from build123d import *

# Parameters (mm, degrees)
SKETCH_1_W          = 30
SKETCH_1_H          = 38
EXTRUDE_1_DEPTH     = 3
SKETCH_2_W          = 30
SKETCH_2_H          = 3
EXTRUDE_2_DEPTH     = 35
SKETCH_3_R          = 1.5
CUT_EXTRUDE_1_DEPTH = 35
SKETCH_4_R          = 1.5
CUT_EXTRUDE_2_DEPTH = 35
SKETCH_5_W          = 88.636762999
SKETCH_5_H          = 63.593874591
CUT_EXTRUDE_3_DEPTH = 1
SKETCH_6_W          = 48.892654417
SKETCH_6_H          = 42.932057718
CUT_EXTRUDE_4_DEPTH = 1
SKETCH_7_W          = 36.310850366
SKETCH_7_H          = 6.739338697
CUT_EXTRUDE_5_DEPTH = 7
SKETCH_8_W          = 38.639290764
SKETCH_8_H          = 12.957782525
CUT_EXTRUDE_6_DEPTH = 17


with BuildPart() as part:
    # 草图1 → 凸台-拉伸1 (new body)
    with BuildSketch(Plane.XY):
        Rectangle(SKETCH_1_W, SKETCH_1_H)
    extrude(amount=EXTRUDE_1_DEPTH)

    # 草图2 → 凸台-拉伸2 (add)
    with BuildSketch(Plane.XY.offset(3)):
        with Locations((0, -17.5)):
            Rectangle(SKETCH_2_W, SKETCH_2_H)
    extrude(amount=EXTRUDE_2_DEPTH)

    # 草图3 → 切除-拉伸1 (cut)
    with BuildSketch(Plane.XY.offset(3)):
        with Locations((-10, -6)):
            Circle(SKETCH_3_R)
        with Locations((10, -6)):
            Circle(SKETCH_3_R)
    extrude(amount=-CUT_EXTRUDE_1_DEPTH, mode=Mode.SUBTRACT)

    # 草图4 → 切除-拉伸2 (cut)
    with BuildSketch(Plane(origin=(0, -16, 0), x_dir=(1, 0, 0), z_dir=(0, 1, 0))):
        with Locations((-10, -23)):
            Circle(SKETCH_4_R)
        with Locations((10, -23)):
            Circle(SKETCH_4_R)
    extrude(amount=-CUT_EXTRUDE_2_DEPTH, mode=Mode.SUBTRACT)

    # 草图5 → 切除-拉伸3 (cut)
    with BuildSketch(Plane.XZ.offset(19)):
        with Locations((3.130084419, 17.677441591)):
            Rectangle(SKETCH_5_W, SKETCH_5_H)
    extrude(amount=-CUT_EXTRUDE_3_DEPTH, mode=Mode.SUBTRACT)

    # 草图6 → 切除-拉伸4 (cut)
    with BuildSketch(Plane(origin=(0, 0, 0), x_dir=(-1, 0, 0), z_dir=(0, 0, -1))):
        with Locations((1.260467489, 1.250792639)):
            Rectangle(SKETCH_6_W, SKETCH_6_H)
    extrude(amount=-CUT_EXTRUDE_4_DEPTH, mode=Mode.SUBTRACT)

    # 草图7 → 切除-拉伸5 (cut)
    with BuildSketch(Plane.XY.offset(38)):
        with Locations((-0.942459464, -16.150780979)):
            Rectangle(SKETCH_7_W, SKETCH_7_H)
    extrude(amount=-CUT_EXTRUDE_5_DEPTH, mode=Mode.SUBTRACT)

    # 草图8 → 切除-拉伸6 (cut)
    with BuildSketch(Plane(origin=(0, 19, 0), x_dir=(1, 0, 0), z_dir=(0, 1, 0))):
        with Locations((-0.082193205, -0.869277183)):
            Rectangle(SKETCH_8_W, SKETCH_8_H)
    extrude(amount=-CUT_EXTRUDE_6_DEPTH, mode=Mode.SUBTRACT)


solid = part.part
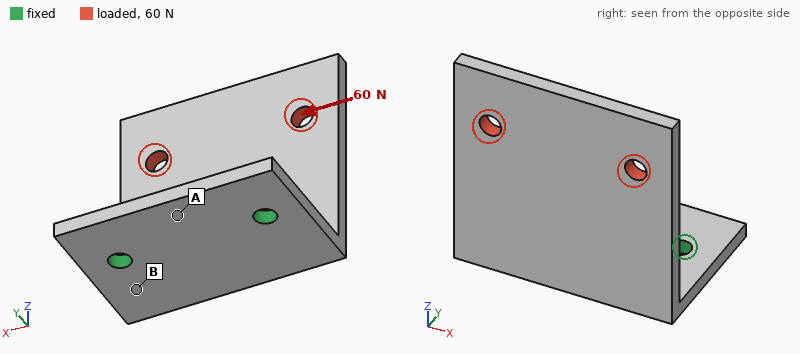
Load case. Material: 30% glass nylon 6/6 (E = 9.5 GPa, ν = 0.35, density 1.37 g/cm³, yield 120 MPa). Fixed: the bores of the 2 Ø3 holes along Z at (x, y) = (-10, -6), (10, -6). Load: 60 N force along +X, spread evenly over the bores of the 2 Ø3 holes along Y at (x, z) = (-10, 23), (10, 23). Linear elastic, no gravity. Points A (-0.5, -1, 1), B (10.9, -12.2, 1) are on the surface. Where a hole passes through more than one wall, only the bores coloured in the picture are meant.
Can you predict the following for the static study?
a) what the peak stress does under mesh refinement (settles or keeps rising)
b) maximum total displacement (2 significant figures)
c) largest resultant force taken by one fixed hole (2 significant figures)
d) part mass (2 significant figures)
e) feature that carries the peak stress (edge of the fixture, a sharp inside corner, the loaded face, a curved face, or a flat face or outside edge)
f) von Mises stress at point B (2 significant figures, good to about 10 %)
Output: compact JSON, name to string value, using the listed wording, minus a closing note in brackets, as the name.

{"what the peak stress does under mesh refinement": "keeps rising", "maximum total displacement": "0.47 mm", "largest resultant force taken by one fixed hole": "72 N", "part mass": "3.9 g", "feature that carries the peak stress": "edge of the fixture", "von Mises stress at point B": "17 MPa"}
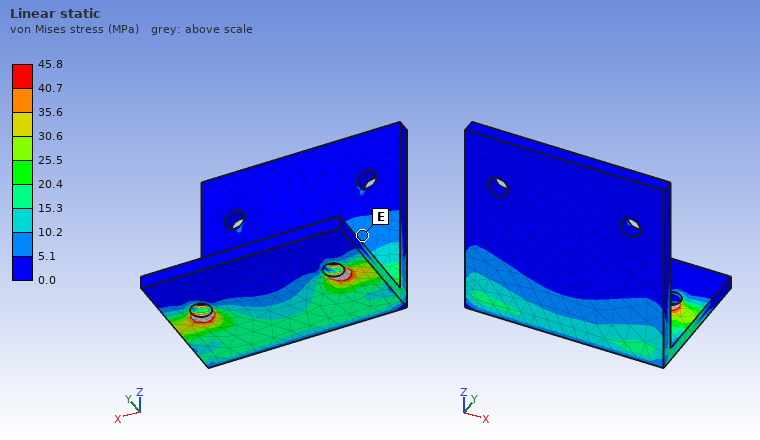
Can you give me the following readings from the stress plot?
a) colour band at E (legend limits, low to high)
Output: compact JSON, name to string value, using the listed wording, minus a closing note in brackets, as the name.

{"colour band at E": "5.1 to 10.2 MPa"}
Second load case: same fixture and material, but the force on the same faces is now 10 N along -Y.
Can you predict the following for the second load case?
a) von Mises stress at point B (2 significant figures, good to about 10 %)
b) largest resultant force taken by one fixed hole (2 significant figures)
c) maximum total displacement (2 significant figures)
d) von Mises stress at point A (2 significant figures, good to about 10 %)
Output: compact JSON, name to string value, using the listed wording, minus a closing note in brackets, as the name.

{"von Mises stress at point B": "9.5 MPa", "largest resultant force taken by one fixed hole": "5.3 N", "maximum total displacement": "0.54 mm", "von Mises stress at point A": "1.7 MPa"}
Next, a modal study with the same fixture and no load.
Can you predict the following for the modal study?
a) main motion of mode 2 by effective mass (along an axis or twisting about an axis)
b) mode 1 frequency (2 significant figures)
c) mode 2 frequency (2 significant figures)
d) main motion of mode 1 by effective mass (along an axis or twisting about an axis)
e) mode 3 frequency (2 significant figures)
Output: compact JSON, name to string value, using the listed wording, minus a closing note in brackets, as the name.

{"main motion of mode 2 by effective mass": "along X", "mode 1 frequency": "670 Hz", "mode 2 frequency": "1600 Hz", "main motion of mode 1 by effective mass": "along Y", "mode 3 frequency": "2400 Hz"}
